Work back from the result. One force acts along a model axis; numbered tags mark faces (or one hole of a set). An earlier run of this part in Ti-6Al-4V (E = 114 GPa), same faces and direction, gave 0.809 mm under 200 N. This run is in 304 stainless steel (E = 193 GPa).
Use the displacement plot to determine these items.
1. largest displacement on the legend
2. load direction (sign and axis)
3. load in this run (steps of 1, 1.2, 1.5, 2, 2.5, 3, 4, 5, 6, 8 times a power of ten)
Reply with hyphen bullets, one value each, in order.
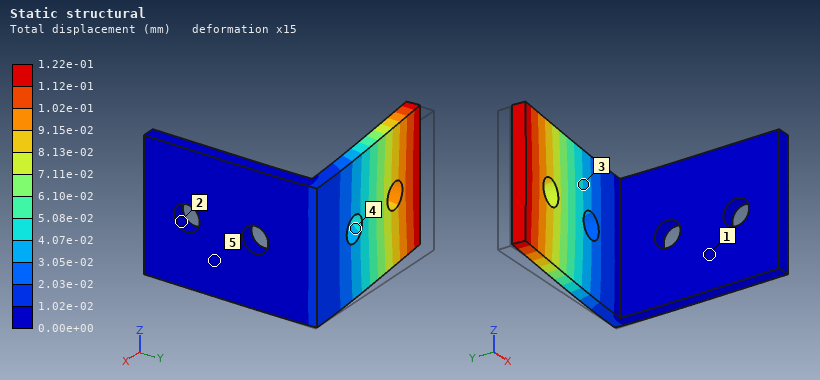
- 1.22e-01 mm
- -Y
- 50 N
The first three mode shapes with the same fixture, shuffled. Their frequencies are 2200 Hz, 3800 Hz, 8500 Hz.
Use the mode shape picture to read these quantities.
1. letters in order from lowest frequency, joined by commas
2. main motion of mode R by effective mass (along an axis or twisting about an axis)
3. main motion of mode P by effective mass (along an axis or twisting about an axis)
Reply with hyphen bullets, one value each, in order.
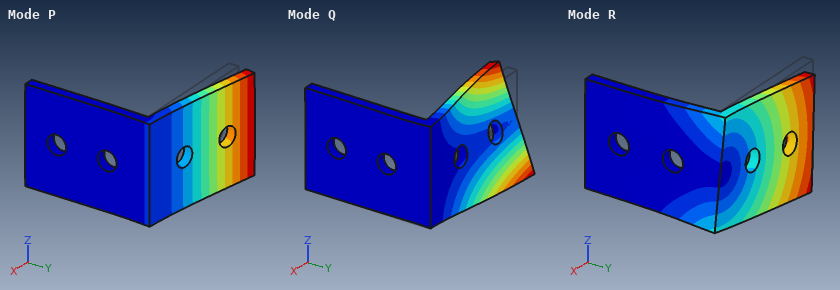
- P, R, Q
- along Z
- along Y
